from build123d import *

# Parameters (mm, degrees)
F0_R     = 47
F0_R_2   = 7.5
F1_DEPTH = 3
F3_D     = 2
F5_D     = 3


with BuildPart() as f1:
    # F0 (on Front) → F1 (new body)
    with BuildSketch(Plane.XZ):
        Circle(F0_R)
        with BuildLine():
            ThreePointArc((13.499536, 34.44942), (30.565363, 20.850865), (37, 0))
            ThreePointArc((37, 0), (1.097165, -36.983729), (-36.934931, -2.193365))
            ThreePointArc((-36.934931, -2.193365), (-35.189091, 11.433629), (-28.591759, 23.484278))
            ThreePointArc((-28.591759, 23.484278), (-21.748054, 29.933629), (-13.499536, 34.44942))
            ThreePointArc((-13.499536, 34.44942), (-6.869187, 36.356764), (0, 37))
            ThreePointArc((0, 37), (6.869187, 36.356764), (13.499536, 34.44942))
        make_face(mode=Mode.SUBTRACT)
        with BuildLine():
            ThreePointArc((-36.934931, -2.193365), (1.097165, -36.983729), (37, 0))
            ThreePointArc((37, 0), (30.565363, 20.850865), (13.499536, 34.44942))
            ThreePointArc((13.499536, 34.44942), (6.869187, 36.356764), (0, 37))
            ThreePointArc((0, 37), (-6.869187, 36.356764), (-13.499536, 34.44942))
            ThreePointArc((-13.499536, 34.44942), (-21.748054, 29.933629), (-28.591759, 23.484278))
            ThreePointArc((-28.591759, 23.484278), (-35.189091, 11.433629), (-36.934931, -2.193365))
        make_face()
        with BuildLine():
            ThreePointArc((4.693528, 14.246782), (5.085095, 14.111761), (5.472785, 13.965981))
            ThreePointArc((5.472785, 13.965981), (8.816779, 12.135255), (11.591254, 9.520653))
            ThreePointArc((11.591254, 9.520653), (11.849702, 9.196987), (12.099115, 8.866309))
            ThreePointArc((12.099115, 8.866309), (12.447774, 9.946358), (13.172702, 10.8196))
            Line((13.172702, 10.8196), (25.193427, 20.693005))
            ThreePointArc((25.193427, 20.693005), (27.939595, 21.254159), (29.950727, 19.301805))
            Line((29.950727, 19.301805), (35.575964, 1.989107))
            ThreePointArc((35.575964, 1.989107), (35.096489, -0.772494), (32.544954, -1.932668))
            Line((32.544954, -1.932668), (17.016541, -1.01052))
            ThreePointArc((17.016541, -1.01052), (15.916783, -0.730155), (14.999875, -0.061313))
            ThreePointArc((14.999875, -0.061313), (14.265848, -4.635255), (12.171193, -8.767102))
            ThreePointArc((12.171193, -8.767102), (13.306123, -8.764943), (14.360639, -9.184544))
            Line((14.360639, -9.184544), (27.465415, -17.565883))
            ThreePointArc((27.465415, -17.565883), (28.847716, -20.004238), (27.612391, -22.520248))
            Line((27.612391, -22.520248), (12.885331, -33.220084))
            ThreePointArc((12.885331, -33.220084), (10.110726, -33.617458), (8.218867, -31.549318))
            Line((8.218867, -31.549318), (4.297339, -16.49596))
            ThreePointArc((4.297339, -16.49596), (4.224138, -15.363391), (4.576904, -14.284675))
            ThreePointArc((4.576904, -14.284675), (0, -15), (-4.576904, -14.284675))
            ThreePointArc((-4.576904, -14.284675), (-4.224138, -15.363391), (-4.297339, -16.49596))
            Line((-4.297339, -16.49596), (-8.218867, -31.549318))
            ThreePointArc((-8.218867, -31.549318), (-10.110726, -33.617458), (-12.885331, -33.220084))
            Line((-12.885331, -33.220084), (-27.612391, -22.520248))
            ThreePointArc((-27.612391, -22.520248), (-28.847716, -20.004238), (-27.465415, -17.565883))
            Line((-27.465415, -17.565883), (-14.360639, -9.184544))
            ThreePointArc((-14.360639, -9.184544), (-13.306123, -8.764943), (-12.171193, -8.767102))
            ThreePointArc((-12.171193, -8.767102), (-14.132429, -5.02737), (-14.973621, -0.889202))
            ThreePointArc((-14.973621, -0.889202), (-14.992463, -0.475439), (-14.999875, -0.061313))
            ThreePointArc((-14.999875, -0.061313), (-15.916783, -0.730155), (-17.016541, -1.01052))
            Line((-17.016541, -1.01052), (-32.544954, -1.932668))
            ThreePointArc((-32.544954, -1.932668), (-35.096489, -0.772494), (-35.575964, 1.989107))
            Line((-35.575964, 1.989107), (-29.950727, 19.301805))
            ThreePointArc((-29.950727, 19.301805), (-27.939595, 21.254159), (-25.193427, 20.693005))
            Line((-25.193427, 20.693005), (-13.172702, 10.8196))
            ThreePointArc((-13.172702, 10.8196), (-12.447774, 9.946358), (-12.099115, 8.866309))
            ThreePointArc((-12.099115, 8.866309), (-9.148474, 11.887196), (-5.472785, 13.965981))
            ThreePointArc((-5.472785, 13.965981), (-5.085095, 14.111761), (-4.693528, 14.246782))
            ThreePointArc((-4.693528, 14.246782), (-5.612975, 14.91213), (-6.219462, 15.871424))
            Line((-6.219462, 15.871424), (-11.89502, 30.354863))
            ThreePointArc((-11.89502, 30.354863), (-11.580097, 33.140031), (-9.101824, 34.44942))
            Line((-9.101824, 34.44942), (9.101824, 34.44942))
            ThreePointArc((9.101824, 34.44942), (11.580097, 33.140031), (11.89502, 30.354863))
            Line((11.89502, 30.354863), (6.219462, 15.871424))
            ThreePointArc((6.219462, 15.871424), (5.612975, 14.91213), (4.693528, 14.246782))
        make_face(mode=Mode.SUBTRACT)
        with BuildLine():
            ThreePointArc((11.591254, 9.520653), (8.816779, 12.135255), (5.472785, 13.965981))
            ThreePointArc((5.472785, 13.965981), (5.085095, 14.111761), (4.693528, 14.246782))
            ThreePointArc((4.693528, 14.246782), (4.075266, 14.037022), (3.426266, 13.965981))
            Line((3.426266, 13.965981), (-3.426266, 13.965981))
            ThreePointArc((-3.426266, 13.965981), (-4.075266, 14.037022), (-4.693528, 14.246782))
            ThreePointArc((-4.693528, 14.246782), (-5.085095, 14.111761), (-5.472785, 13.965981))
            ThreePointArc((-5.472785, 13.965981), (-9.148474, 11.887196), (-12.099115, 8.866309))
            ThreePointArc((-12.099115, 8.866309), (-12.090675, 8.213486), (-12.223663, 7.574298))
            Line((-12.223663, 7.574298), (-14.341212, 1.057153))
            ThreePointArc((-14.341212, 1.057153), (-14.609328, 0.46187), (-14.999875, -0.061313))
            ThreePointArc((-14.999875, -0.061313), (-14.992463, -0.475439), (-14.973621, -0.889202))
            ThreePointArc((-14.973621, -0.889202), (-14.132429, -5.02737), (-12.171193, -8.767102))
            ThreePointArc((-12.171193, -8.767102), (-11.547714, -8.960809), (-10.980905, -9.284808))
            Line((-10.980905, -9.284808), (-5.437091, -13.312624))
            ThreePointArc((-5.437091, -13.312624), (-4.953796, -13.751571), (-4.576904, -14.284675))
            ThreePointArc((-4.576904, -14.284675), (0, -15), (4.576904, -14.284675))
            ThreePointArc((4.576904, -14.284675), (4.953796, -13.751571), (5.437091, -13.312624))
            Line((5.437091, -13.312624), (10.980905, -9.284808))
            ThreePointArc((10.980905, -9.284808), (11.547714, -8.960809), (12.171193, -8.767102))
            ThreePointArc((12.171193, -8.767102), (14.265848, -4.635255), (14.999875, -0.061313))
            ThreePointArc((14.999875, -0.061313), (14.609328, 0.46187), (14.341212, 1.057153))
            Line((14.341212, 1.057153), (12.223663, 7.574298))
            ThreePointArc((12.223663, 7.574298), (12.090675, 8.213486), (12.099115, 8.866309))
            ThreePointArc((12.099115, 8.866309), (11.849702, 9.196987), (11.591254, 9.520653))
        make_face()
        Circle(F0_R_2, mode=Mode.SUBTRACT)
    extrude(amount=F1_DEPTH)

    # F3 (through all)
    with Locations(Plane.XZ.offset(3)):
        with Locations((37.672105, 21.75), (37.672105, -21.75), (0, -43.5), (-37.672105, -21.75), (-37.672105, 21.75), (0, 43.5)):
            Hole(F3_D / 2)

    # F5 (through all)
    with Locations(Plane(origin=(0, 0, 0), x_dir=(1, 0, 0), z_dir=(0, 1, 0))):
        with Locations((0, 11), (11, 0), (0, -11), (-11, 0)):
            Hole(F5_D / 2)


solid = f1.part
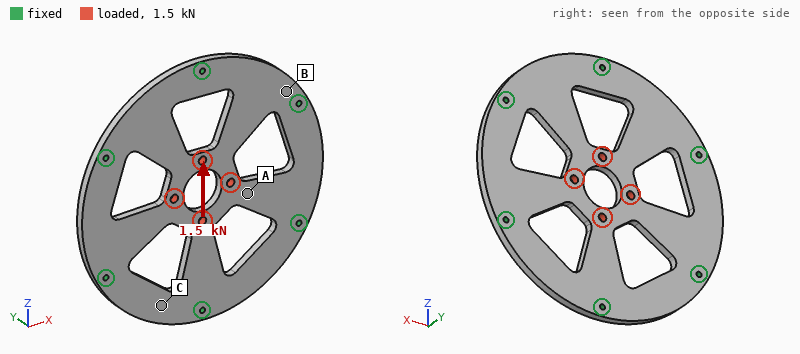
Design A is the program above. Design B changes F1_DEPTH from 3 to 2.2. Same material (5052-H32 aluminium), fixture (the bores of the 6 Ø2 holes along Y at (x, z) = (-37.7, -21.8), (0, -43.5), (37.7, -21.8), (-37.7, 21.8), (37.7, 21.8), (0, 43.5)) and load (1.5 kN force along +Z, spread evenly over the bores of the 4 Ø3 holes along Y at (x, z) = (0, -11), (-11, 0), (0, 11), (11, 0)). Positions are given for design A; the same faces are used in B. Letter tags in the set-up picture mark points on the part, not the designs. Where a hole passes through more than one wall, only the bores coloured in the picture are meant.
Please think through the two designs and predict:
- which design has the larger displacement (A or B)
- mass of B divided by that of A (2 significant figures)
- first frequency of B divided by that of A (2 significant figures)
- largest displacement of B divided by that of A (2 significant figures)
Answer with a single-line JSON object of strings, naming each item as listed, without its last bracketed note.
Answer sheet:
{"which design has the larger displacement": "B", "mass of B divided by that of A": "0.73", "first frequency of B divided by that of A": "0.76", "largest displacement of B divided by that of A": "1.4"}
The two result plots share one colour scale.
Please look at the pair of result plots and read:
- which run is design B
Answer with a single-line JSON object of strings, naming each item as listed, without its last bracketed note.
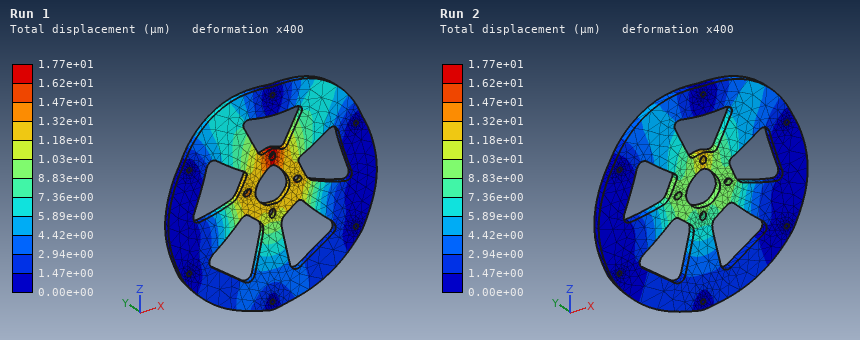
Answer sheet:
{"which run is design B": "Run 1"}
